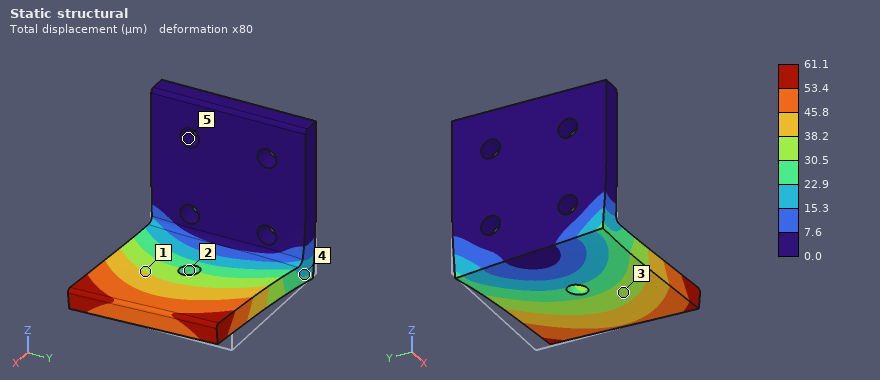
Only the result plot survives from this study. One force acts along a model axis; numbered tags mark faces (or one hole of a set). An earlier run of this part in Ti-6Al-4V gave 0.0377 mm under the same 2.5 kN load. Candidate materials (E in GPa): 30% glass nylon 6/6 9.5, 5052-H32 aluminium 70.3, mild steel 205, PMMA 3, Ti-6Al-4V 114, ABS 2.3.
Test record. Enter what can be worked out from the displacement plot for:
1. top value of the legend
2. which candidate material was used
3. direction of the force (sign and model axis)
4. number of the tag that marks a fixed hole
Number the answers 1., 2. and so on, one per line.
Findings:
1. 61.1 µm
2. 5052-H32 aluminium
3. -Y
4. 5
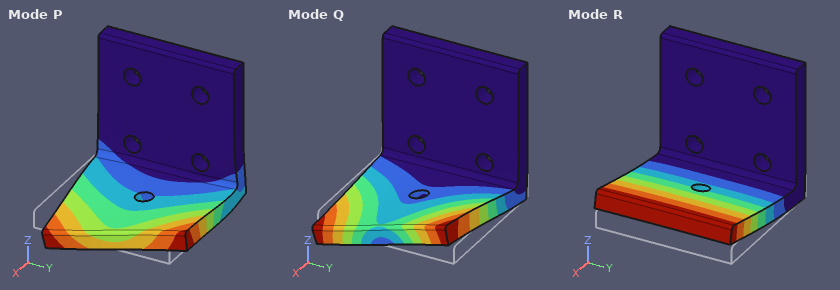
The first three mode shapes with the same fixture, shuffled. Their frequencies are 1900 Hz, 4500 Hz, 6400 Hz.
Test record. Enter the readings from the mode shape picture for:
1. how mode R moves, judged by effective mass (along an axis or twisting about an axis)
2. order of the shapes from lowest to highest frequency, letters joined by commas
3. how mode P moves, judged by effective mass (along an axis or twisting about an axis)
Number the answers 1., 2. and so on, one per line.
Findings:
1. along Z
2. R, Q, P
3. along Y
